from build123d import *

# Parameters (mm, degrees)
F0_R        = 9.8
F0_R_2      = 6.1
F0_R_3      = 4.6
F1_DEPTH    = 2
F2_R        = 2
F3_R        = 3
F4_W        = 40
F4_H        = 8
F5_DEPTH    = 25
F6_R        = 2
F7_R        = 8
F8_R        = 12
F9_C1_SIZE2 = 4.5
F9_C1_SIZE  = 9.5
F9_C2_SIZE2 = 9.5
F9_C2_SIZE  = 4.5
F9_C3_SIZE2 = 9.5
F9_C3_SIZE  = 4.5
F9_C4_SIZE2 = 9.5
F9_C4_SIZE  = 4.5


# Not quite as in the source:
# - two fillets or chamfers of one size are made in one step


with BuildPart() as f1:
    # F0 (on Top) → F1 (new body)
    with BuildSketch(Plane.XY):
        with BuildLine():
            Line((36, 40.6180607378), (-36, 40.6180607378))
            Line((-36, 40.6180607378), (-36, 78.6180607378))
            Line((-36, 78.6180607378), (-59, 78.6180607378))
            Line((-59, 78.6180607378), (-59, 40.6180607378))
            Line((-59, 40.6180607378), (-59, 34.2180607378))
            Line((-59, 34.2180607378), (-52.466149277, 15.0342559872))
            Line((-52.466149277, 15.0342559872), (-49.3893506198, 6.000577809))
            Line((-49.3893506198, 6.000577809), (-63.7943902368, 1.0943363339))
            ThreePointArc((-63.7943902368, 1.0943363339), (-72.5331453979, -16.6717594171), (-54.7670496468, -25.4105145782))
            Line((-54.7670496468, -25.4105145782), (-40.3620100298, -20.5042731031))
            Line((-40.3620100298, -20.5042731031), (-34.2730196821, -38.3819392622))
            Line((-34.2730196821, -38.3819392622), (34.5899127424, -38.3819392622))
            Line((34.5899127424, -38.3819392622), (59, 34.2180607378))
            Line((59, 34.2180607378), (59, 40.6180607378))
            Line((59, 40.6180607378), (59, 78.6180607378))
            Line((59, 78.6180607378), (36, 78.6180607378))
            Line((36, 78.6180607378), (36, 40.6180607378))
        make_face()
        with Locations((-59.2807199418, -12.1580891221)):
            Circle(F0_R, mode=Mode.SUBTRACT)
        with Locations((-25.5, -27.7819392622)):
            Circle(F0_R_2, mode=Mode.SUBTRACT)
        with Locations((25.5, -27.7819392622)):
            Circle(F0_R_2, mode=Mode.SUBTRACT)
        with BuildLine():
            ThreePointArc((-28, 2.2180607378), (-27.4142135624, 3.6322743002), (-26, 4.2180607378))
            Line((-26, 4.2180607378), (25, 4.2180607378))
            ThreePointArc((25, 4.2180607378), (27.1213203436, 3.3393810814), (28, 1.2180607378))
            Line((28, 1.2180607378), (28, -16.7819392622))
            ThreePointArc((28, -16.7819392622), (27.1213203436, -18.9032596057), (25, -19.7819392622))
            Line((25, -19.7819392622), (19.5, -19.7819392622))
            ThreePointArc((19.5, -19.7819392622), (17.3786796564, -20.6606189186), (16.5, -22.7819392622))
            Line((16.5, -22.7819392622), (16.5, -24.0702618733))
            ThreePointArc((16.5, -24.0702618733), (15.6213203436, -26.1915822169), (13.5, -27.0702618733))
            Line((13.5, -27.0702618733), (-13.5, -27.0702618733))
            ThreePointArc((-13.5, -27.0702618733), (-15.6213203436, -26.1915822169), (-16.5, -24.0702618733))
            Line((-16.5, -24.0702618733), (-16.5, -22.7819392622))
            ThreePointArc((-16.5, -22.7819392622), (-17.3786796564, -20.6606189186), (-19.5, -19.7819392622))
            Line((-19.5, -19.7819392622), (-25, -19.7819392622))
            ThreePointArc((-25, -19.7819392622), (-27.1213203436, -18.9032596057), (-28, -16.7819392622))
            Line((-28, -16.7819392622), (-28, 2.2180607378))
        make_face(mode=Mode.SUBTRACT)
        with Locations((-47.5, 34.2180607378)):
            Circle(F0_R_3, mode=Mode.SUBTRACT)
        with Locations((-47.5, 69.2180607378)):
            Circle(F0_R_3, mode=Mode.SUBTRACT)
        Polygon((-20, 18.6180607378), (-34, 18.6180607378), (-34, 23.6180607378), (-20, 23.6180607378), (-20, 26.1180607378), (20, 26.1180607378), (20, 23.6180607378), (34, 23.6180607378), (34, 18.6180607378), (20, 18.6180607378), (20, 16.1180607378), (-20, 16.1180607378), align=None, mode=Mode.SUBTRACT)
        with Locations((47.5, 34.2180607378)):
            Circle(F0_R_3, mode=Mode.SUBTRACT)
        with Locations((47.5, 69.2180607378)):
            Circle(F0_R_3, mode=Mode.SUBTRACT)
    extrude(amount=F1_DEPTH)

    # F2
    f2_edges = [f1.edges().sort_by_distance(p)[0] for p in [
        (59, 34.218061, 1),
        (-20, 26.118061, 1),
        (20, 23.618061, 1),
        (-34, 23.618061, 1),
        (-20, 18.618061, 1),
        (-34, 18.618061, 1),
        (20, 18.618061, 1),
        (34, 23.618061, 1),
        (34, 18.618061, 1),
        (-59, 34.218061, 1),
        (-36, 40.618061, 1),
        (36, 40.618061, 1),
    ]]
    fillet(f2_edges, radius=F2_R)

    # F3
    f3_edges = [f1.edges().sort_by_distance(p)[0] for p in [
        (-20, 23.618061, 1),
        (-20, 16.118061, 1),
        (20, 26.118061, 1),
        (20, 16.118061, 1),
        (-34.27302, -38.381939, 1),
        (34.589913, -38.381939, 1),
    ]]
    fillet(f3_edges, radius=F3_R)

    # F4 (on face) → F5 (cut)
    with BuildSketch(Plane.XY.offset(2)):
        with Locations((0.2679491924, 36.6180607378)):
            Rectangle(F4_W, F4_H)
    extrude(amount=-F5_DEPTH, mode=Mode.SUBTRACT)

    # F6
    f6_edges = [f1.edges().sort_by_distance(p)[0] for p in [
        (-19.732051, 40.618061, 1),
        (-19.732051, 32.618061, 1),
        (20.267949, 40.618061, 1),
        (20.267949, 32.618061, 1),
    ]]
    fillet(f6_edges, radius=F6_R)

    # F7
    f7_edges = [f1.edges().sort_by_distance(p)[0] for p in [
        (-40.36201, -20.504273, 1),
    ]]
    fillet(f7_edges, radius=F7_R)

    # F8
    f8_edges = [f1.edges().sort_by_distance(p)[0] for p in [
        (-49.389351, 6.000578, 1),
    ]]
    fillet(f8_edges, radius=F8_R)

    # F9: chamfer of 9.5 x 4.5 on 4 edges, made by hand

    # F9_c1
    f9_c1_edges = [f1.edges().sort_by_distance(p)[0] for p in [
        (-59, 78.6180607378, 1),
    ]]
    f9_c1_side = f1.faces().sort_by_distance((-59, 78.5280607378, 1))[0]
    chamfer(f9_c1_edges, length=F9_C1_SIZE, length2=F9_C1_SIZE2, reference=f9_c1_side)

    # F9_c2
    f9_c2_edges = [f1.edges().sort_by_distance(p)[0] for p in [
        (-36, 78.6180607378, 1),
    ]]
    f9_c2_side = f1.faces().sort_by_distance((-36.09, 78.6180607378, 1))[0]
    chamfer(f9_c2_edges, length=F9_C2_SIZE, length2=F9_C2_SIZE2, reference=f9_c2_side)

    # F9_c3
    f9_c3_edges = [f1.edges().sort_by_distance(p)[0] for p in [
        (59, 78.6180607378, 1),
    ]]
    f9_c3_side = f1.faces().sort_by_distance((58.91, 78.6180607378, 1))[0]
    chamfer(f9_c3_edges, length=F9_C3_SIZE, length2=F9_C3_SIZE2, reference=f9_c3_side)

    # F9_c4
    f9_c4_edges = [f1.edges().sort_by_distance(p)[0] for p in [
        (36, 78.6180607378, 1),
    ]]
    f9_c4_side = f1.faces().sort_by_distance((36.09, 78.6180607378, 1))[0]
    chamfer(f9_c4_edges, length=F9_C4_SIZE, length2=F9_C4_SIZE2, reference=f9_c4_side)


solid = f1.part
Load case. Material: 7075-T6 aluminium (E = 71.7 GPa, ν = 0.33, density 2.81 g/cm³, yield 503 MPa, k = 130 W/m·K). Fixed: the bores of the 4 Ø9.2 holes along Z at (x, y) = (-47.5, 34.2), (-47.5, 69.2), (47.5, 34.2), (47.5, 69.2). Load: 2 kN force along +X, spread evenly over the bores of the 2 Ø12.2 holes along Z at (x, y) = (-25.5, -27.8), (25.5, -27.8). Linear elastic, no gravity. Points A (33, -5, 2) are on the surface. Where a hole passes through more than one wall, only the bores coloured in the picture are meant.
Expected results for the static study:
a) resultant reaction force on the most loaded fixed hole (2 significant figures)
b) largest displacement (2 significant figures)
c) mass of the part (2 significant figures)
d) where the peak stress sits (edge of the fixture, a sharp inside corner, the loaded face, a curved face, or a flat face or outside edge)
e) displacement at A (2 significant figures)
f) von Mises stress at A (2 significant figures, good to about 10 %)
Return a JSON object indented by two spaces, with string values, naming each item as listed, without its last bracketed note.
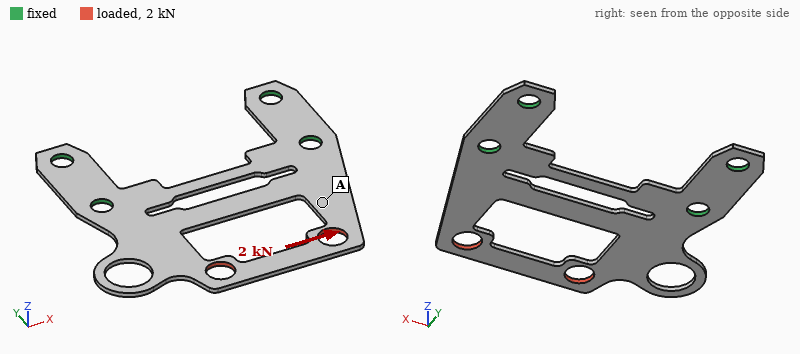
{
  "resultant reaction force on the most loaded fixed hole": "1.6 kN",
  "largest displacement": "0.32 mm",
  "mass of the part": "38 g",
  "where the peak stress sits": "a curved face",
  "displacement at A": "0.15 mm",
  "von Mises stress at A": "52 MPa"
}
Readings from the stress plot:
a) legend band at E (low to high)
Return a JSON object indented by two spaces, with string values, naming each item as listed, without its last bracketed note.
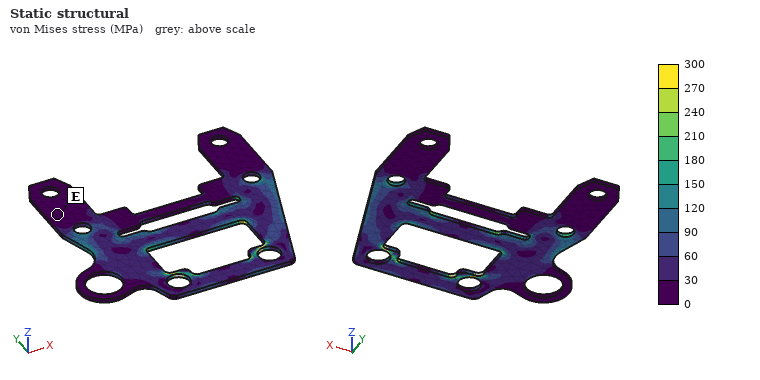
{
  "legend band at E": "0 to 30 MPa"
}
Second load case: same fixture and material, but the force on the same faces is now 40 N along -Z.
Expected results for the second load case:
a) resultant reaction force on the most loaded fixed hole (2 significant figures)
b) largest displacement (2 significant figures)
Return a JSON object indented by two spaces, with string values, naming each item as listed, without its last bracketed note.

{
  "resultant reaction force on the most loaded fixed hole": "21 N",
  "largest displacement": "1.8 mm"
}
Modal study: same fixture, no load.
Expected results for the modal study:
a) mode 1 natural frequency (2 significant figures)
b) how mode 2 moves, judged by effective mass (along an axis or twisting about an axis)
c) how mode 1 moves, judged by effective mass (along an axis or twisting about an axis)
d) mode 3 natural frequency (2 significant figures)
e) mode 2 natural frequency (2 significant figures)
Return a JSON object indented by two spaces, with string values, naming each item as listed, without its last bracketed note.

{
  "mode 1 natural frequency": "300 Hz",
  "how mode 2 moves, judged by effective mass": "twisting about Y",
  "how mode 1 moves, judged by effective mass": "along Z",
  "mode 3 natural frequency": "1100 Hz",
  "mode 2 natural frequency": "630 Hz"
}
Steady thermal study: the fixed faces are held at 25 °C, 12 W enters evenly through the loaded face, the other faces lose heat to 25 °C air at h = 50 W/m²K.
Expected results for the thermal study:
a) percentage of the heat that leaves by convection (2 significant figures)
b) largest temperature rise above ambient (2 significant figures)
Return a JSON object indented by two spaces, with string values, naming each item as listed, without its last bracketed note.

{
  "percentage of the heat that leaves by convection": "67 %",
  "largest temperature rise above ambient": "46 K"
}
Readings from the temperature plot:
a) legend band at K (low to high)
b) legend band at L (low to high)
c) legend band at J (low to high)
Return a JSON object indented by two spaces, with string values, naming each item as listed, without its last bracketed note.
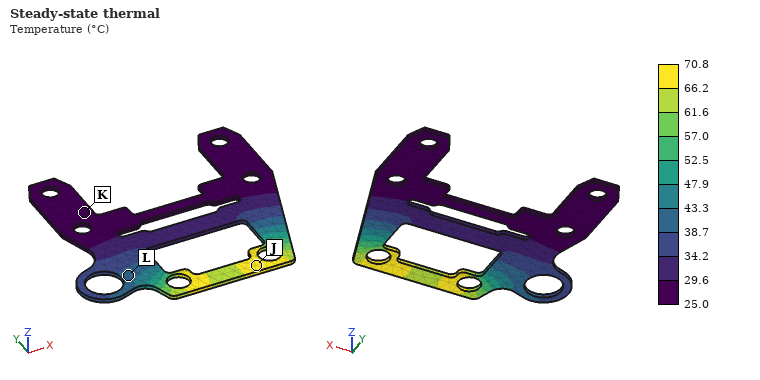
{
  "legend band at K": "25.0 to 29.6 °C",
  "legend band at L": "38.7 to 43.3 °C",
  "legend band at J": "66.2 to 70.8 °C"
}
